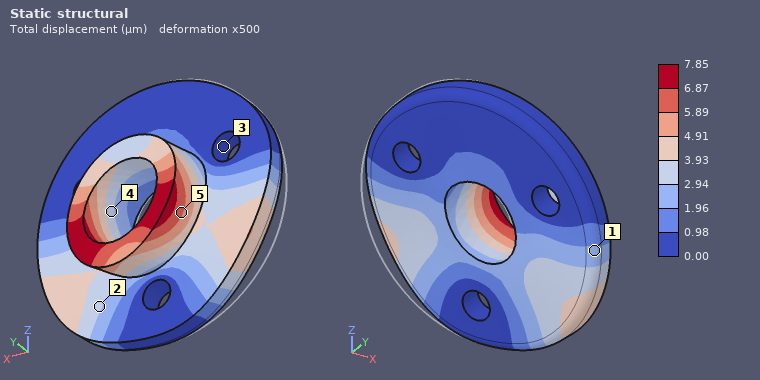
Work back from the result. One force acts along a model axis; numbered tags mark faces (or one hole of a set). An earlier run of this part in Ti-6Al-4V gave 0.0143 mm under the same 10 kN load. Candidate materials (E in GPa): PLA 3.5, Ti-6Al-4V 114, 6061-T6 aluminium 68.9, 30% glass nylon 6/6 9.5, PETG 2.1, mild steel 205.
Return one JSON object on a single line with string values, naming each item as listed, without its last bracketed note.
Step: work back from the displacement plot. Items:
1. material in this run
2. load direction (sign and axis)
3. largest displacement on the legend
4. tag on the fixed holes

{"material in this run": "mild steel", "load direction": "+X", "largest displacement on the legend": "7.85 µm", "tag on the fixed holes": "3"}
